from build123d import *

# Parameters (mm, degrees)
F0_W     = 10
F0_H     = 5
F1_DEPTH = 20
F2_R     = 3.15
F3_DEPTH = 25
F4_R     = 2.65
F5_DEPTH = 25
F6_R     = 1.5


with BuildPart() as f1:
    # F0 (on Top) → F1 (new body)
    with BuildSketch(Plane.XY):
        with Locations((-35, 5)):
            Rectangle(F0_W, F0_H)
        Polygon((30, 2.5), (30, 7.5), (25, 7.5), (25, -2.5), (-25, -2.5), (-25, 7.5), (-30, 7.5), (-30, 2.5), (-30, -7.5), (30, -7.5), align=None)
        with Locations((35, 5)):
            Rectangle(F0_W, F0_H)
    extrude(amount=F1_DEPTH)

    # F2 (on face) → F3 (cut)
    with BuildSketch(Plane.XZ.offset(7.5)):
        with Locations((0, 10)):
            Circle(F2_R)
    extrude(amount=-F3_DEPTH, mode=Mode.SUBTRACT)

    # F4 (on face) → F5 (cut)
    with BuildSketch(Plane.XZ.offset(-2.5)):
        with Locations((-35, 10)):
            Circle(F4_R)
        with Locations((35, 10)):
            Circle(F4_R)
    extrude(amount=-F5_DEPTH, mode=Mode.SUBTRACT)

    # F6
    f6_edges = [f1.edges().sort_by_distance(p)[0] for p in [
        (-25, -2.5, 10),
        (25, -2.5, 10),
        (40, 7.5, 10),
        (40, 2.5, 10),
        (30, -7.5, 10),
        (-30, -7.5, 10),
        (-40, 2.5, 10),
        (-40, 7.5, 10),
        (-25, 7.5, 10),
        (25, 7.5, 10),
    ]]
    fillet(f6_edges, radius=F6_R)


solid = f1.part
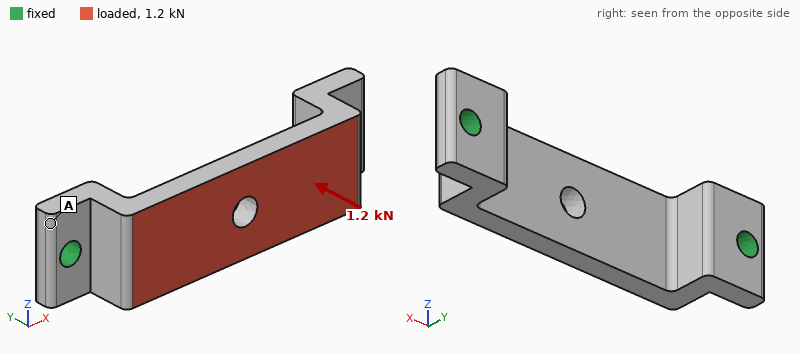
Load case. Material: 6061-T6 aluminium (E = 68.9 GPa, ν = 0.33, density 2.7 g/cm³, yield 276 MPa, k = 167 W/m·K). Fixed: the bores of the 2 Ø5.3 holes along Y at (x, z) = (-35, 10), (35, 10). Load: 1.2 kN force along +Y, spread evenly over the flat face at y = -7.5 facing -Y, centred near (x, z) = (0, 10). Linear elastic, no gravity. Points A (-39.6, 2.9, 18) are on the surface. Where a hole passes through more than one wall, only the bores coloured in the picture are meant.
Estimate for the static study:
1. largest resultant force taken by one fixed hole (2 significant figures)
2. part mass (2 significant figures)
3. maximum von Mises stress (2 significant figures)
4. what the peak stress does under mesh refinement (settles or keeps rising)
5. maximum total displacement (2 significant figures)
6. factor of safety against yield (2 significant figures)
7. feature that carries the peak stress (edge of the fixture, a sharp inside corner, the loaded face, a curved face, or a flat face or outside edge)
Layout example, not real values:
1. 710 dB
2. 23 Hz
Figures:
1. 940 N
2. 26 g
3. 87 MPa
4. settles
5. 50 µm
6. 3.2
7. the loaded face
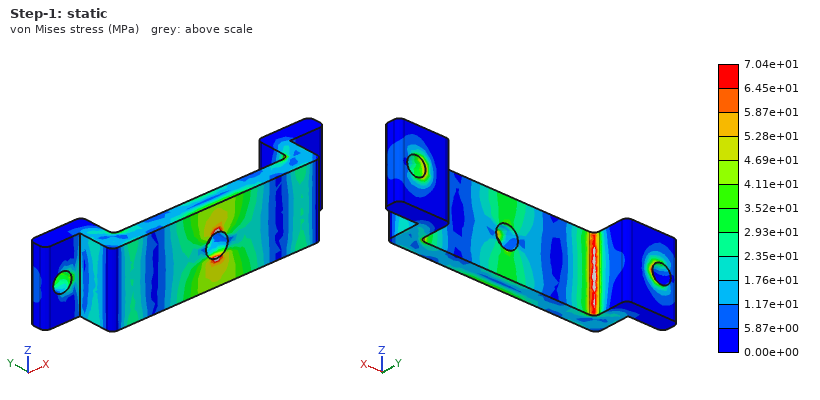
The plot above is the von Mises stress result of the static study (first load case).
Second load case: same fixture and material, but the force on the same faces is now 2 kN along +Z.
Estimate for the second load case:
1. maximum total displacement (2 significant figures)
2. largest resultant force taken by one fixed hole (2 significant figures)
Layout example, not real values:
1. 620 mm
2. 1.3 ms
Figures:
1. 83 µm
2. 1.0 kN
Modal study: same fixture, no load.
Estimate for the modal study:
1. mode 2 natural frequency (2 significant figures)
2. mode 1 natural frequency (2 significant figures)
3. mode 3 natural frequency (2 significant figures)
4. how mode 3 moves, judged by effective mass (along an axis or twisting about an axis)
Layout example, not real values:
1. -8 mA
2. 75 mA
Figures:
1. 7500 Hz
2. 7400 Hz
3. 9100 Hz
4. along X
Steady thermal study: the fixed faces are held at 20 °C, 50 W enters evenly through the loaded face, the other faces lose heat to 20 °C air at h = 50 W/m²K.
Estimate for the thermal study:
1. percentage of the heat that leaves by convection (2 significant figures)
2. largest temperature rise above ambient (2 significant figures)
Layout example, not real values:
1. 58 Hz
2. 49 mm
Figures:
1. 7.0 %
2. 37 K
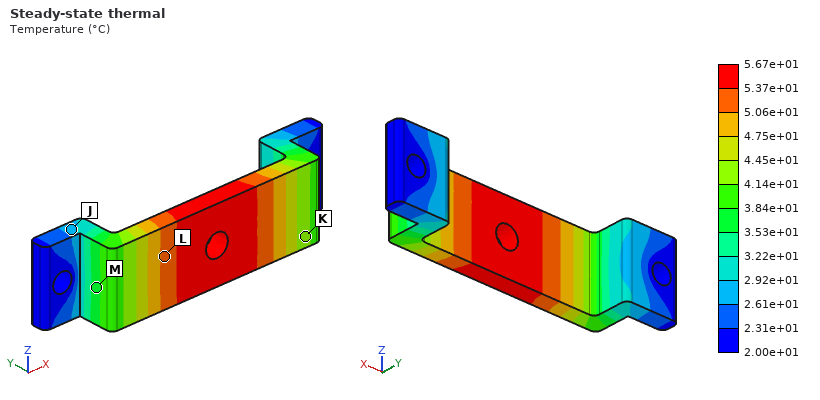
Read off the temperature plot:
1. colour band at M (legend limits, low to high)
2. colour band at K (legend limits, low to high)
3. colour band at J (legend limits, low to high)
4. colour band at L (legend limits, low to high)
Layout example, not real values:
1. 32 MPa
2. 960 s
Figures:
1. 3.53e+01 to 3.84e+01 °C
2. 4.14e+01 to 4.45e+01 °C
3. 2.61e+01 to 2.92e+01 °C
4. 5.06e+01 to 5.37e+01 °C
